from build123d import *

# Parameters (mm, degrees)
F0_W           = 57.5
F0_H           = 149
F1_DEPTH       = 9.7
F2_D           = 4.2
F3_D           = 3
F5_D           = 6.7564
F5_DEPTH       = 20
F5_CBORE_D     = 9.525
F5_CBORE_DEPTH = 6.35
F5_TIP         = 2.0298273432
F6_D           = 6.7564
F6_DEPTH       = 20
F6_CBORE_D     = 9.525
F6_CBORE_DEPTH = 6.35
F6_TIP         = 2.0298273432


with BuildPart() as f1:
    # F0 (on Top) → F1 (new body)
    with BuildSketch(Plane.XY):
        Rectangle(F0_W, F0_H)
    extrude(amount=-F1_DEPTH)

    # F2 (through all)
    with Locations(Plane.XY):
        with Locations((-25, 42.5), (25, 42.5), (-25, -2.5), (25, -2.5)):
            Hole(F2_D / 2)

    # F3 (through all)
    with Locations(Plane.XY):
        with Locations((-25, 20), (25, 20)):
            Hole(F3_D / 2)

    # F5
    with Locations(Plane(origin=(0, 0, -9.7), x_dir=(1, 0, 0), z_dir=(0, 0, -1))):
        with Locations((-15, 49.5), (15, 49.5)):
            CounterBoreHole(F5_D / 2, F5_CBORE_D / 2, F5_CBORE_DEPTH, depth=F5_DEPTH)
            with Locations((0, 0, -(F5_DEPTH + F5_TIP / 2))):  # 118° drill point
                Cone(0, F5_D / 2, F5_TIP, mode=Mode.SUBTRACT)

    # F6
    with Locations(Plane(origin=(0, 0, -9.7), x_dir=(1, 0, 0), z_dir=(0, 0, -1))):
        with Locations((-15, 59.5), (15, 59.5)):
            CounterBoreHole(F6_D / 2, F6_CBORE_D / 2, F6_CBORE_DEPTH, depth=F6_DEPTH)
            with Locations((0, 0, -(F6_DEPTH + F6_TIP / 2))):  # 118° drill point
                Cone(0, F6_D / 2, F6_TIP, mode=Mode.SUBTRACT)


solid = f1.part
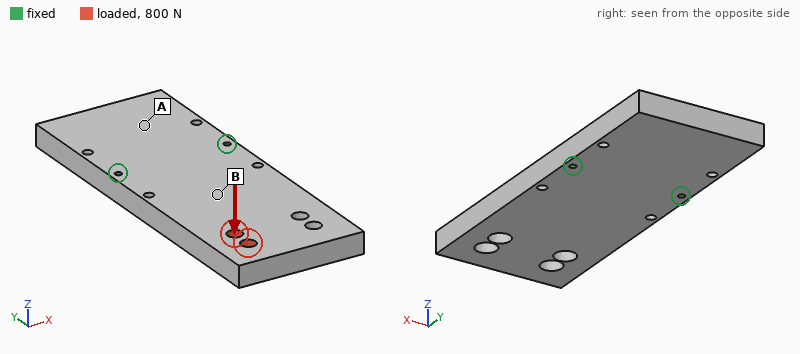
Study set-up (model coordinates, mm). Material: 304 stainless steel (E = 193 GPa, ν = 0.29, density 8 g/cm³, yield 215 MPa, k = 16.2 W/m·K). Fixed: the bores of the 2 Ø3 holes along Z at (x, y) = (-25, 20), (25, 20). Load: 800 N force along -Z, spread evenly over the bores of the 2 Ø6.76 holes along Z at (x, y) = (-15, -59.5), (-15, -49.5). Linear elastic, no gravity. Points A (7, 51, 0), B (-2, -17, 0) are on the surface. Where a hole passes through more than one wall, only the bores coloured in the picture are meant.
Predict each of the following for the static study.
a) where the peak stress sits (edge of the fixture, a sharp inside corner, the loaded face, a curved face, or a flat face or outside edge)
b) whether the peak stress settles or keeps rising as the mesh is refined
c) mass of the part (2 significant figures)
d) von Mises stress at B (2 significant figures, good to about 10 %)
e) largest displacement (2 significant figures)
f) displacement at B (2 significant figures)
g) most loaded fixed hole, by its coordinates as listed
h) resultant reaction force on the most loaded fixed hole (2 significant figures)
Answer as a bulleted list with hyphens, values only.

- edge of the fixture
- keeps rising
- 640 g
- 38 MPa
- 0.27 mm
- 0.067 mm
- (-25, 20)
- 650 N
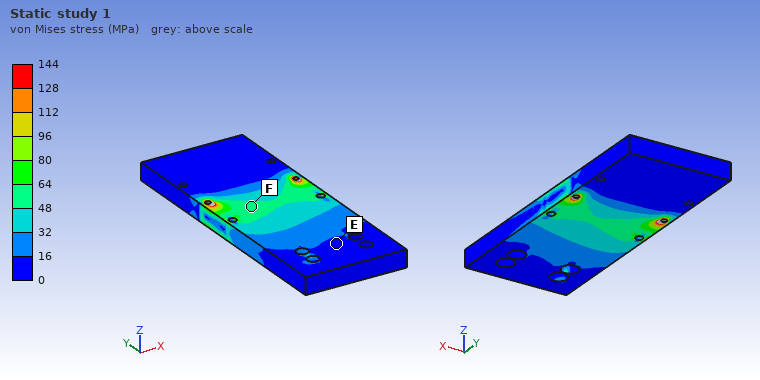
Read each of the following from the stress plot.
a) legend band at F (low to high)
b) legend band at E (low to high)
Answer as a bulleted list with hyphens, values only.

- 48 to 64 MPa
- 0 to 16 MPa
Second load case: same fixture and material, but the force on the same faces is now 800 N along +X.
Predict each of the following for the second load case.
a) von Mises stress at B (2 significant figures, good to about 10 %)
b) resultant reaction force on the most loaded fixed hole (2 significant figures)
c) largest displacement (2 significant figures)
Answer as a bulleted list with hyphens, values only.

- 6.4 MPa
- 1.3 kN
- 10 µm
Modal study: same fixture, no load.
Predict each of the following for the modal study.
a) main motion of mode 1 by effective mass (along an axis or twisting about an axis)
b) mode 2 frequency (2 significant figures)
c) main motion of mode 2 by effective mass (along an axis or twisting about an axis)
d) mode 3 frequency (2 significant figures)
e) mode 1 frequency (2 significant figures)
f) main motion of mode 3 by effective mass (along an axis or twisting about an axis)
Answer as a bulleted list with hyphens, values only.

- along Z
- 2100 Hz
- along Z
- 2900 Hz
- 750 Hz
- twisting about Y
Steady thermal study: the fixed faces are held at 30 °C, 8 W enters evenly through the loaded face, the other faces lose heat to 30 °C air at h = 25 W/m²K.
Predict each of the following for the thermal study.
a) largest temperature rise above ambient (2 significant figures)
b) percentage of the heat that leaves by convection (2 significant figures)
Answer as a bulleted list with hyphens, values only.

- 52 K
- 77 %
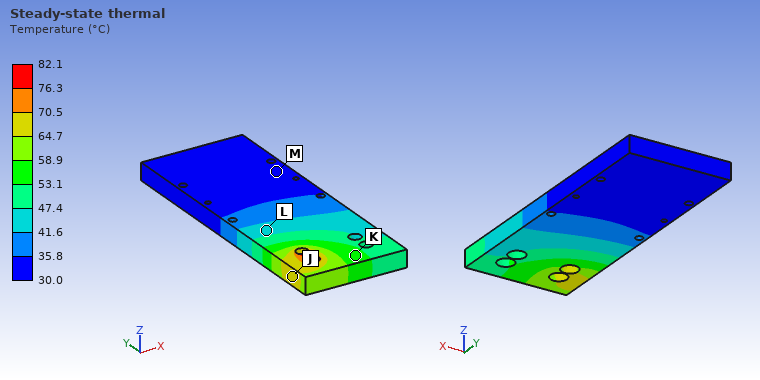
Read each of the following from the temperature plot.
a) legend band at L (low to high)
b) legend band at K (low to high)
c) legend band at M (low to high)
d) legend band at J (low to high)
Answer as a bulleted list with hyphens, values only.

- 41.6 to 47.4 °C
- 53.1 to 58.9 °C
- 30.0 to 35.8 °C
- 64.7 to 70.5 °C
